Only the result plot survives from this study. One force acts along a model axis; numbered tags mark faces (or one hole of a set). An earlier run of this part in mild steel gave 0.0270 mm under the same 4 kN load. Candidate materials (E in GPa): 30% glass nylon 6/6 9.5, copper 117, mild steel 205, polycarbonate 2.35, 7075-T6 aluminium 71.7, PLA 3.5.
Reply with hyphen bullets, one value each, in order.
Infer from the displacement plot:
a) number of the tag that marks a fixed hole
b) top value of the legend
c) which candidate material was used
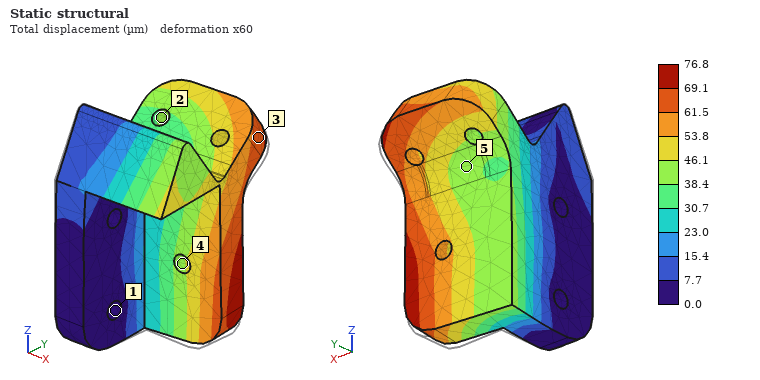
- 1
- 76.8 µm
- 7075-T6 aluminium
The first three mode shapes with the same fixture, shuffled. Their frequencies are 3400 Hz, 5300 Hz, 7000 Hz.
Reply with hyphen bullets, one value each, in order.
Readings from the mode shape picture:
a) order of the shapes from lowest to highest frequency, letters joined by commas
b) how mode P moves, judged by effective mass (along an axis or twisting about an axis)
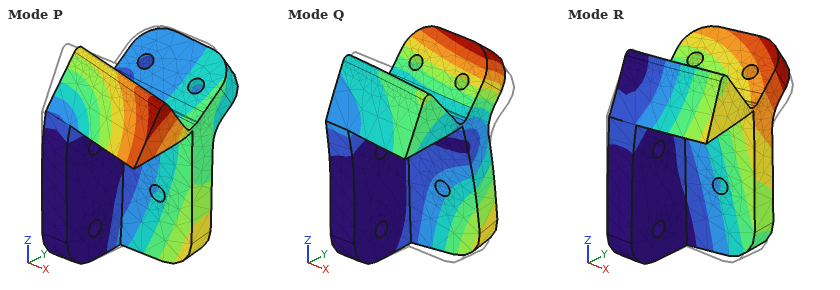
- R, P, Q
- along Z
